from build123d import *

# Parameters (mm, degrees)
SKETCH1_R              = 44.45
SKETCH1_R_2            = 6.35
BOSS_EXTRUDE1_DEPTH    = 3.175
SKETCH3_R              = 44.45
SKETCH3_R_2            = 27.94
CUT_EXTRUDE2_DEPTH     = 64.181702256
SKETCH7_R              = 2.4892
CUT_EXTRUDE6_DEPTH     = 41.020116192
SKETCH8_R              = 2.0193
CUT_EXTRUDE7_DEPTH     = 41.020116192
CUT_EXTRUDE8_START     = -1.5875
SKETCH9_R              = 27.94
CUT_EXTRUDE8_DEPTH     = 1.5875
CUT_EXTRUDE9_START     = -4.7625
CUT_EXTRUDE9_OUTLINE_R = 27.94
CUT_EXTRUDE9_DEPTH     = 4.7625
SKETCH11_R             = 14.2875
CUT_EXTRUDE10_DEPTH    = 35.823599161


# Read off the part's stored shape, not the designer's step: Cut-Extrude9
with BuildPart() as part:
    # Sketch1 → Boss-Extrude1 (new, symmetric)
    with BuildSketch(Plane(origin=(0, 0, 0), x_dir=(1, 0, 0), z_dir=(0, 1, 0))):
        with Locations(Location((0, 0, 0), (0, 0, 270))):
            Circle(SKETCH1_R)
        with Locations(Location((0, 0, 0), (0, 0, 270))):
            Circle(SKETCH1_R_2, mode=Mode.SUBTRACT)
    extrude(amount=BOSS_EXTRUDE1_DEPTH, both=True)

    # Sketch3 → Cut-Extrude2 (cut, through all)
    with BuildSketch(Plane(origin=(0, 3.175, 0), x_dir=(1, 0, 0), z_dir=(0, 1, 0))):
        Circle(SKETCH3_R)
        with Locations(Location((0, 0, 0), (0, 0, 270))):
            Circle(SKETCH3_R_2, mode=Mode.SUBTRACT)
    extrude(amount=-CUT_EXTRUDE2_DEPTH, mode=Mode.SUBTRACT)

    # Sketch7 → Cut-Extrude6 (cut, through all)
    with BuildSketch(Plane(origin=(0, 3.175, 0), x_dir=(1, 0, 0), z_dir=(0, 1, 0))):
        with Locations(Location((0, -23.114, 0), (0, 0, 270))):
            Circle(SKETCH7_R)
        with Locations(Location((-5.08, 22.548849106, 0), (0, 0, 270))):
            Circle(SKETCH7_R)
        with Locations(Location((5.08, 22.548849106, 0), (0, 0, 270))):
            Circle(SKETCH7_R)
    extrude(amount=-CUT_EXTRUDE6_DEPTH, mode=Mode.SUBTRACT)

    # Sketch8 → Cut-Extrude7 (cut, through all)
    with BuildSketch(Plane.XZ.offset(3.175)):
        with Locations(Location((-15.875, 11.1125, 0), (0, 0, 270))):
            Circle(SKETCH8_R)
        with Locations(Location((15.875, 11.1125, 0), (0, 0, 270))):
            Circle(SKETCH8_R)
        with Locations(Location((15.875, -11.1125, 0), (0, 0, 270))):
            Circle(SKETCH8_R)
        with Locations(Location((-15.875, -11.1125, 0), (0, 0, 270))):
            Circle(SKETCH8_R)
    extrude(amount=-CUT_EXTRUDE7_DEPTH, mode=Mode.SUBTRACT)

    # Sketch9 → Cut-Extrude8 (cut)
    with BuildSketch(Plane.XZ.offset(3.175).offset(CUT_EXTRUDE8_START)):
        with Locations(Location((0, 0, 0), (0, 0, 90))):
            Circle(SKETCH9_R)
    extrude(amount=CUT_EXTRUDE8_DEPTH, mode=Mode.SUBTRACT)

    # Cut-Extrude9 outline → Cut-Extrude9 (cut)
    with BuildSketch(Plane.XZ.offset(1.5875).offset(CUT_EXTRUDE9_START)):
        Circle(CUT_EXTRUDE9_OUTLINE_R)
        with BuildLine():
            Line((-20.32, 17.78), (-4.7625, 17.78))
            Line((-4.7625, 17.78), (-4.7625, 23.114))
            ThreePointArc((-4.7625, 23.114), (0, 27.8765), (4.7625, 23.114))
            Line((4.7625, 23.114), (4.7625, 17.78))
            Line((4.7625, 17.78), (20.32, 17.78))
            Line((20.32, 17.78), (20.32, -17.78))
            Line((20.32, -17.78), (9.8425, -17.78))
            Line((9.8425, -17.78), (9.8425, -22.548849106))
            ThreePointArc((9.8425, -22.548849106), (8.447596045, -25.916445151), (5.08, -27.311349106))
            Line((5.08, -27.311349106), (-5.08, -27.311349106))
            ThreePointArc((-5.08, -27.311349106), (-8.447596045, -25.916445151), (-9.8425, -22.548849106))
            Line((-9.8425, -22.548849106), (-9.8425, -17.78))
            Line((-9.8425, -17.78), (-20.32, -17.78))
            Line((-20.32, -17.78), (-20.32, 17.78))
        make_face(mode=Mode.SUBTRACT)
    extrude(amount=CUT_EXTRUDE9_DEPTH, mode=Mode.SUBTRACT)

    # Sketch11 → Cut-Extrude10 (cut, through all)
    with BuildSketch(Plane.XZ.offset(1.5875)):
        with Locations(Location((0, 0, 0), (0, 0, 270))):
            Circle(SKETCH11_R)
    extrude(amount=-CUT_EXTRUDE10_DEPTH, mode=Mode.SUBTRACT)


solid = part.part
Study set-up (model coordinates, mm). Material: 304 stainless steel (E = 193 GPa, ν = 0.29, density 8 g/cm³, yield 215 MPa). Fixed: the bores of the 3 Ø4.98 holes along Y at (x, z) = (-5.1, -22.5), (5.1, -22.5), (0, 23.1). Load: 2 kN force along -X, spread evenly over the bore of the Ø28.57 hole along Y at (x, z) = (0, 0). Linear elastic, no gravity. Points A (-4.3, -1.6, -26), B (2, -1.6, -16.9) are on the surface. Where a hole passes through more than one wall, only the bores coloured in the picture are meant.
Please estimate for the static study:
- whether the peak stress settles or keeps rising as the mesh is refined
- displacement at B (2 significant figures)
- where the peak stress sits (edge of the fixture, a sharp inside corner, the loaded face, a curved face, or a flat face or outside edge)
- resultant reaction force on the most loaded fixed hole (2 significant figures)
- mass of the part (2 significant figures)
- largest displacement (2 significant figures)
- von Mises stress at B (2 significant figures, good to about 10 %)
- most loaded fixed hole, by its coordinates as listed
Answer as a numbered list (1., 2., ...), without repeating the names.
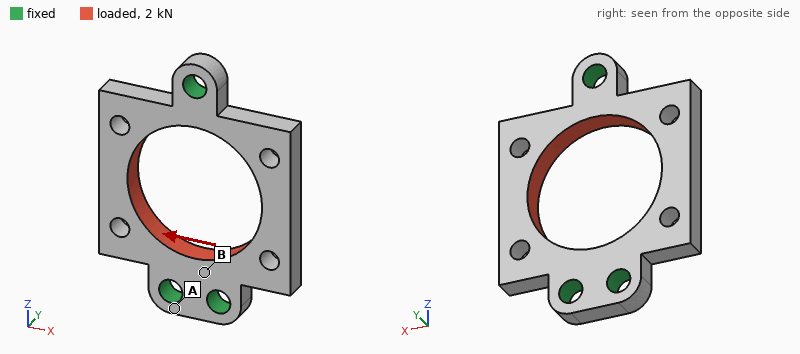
1. keeps rising
2. 0.61 µm
3. edge of the fixture
4. 1.0 kN
5. 37 g
6. 3.8 µm
7. 20 MPa
8. (0, 23.1)
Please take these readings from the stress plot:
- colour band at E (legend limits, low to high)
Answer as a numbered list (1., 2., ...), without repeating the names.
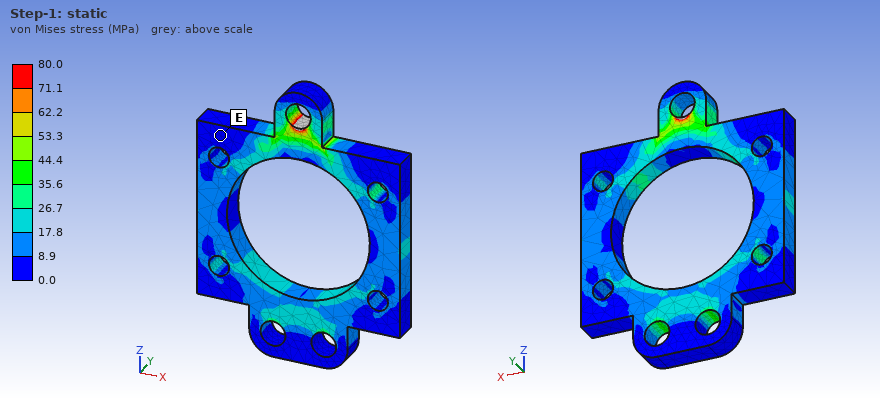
1. 0.0 to 8.9 MPa
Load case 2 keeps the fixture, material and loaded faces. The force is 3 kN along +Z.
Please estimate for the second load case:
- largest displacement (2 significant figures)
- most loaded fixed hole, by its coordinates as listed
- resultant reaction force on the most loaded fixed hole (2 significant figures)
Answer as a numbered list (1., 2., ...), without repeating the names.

1. 5.7 µm
2. (0, 23.1)
3. 1.2 kN
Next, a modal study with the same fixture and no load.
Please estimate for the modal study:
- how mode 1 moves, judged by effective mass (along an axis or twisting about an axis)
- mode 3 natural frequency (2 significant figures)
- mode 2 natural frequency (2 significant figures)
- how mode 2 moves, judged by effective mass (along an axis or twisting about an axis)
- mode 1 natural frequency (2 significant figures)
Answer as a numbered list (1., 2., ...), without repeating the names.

1. twisting about Z
2. 13 kHz
3. 6100 Hz
4. along Y
5. 5500 Hz
